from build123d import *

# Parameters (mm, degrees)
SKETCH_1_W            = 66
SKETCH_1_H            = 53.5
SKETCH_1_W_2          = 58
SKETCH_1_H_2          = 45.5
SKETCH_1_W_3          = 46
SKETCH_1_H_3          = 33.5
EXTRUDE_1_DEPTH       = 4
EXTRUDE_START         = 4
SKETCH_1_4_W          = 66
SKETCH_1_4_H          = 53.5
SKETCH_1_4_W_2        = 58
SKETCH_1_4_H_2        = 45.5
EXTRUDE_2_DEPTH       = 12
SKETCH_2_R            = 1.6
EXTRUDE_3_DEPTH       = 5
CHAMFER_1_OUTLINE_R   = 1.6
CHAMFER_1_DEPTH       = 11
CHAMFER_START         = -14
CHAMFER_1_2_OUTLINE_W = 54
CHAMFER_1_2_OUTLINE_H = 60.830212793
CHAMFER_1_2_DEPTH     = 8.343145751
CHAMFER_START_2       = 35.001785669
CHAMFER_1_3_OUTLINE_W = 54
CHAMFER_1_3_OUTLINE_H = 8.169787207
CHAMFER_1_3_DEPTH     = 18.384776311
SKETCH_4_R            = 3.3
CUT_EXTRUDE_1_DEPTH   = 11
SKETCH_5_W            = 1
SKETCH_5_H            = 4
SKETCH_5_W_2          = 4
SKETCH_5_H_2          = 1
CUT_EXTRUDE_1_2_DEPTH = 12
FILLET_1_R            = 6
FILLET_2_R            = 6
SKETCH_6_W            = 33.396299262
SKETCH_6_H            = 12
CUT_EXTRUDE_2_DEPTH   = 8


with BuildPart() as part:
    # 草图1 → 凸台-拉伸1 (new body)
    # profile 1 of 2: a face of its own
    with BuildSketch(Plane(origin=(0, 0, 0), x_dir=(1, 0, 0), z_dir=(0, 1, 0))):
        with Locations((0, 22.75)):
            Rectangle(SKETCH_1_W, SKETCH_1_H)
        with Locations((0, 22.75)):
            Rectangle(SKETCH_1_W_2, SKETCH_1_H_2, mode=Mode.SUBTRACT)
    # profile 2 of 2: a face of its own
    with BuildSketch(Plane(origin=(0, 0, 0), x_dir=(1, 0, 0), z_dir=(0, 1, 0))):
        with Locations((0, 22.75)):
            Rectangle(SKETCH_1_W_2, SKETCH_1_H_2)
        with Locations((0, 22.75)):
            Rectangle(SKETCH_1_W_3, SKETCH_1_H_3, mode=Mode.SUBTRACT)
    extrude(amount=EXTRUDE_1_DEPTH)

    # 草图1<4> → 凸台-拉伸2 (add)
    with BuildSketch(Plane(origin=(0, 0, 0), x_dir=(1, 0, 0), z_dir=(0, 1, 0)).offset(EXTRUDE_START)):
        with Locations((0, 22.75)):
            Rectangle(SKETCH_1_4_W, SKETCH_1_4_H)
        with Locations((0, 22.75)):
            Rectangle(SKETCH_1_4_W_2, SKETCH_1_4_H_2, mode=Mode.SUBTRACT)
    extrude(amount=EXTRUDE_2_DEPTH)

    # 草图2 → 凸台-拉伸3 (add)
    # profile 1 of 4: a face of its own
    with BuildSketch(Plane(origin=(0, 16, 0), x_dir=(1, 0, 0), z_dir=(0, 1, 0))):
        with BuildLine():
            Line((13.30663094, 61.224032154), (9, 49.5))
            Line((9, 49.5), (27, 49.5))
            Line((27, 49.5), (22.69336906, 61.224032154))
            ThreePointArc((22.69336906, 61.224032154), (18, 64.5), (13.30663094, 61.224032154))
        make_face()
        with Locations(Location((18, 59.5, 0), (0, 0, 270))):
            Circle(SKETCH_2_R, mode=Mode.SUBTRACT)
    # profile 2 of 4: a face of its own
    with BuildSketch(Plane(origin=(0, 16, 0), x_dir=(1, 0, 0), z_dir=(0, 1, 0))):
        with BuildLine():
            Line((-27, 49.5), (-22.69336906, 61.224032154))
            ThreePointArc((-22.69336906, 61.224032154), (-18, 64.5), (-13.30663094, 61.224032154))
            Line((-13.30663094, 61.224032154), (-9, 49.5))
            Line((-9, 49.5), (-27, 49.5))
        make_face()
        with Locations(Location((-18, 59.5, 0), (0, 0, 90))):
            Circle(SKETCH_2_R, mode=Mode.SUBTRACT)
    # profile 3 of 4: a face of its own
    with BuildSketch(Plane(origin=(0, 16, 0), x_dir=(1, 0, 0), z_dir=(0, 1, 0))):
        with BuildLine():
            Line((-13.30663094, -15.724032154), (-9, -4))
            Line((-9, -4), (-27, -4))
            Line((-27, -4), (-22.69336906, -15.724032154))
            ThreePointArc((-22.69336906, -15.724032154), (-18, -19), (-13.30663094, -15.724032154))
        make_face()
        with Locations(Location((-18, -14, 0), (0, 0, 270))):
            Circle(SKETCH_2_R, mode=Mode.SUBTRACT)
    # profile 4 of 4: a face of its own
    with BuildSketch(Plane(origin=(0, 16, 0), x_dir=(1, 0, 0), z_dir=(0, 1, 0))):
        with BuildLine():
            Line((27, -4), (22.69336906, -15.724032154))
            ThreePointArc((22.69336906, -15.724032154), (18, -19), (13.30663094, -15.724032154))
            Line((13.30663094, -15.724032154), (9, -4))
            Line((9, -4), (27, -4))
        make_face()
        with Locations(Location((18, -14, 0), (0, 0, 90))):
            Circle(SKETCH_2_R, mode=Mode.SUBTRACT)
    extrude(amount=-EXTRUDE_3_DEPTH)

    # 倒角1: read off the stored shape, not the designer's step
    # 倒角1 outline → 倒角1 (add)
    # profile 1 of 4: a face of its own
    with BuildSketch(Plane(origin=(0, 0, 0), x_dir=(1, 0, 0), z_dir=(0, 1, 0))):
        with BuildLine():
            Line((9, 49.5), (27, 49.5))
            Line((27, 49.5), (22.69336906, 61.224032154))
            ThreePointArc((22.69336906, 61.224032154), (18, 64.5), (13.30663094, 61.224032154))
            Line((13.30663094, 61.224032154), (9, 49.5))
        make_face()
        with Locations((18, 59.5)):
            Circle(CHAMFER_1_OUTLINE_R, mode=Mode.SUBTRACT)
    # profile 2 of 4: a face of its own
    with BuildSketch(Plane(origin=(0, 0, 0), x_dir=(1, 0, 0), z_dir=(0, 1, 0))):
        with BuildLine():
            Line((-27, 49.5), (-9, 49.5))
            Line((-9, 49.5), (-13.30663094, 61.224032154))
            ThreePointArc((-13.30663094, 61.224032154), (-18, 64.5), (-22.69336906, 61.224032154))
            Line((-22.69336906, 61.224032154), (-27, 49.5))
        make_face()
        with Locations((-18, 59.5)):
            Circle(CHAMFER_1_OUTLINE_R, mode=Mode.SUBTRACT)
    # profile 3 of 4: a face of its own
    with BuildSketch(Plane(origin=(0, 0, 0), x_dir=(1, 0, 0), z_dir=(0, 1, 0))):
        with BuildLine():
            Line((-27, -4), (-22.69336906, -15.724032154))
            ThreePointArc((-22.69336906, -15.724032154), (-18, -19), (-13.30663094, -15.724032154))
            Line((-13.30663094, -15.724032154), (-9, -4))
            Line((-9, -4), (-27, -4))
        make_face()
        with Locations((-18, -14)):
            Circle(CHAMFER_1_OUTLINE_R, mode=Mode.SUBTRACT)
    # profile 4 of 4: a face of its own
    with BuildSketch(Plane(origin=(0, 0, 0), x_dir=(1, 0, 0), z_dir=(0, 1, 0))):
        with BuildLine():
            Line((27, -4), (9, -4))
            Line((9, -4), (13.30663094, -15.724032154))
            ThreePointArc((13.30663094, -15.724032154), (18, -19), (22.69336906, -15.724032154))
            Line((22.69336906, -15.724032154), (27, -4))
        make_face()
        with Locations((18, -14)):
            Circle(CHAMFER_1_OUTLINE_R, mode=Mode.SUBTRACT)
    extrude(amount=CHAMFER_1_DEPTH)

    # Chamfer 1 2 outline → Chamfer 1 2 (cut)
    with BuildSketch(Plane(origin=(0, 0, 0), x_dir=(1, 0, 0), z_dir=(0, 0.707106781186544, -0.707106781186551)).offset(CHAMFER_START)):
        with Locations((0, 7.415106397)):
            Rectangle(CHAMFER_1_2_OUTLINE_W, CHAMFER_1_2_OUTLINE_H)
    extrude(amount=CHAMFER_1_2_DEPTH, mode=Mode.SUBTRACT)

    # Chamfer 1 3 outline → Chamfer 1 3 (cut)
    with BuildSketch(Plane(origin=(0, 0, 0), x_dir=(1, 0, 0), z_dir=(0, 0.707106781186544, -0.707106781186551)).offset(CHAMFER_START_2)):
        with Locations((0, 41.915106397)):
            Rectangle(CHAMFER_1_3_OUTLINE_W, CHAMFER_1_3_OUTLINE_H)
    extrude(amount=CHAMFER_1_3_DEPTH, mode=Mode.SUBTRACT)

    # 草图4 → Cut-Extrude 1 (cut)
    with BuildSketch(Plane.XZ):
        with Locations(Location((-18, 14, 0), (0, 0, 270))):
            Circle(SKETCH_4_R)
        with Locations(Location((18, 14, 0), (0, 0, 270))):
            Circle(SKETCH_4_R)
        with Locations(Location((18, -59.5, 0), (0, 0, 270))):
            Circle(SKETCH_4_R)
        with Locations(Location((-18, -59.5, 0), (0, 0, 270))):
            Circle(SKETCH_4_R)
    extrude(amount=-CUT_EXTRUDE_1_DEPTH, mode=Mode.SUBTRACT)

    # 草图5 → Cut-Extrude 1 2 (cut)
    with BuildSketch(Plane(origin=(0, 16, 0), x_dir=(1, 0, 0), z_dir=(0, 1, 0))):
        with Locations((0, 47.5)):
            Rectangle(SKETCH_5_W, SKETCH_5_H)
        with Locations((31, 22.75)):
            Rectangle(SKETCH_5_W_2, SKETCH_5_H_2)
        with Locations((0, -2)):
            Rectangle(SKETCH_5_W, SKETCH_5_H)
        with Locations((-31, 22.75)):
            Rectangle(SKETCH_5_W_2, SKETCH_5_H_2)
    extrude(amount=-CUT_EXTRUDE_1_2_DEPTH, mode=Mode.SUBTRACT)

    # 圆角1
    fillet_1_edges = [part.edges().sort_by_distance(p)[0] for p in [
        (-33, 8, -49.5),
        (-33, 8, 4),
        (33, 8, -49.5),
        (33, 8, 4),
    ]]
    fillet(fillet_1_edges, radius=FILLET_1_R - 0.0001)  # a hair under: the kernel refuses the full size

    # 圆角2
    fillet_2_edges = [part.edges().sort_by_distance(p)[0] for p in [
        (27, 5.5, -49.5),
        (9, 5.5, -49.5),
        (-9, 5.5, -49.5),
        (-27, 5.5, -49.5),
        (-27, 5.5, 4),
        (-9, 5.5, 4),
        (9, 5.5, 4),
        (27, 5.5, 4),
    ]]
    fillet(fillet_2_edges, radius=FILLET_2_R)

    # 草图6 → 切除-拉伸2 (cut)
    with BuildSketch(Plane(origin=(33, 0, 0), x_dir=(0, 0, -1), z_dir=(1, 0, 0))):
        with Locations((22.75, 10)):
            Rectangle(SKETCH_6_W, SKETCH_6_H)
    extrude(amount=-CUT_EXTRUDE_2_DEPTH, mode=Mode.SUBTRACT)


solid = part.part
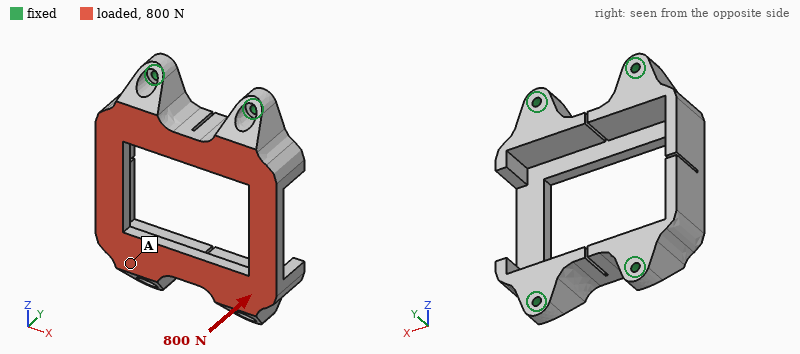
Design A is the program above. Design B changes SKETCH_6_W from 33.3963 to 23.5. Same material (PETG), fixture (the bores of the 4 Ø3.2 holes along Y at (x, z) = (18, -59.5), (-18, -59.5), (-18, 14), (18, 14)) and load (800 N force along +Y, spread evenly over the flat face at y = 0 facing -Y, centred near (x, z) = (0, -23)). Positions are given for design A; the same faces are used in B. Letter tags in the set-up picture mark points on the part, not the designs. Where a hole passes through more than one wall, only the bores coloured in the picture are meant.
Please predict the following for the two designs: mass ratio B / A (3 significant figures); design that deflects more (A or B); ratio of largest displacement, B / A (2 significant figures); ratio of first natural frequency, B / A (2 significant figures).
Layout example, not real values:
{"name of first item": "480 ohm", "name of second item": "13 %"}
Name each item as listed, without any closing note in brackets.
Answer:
{"mass ratio B / A": "1.02", "design that deflects more": "A", "ratio of largest displacement, B / A": "0.86", "ratio of first natural frequency, B / A": "1.00"}
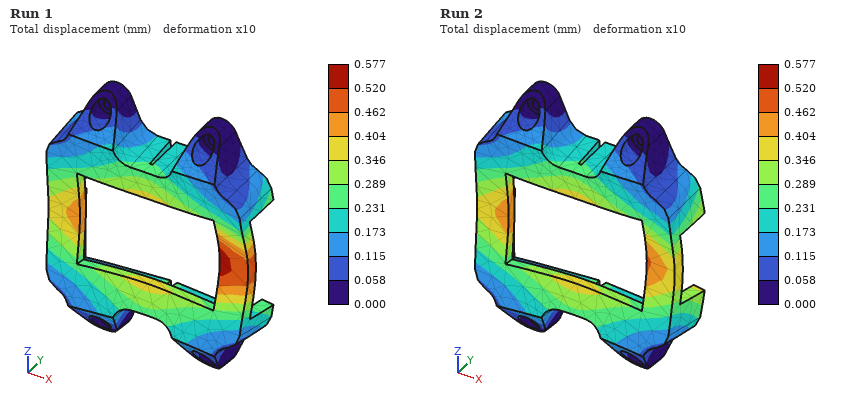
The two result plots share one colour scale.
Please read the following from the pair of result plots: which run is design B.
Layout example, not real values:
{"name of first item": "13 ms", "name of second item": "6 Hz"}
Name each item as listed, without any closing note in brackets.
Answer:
{"which run is design B": "Run 2"}
